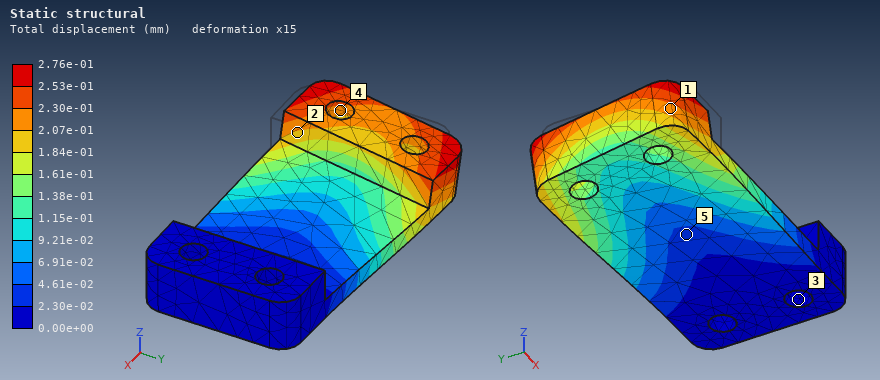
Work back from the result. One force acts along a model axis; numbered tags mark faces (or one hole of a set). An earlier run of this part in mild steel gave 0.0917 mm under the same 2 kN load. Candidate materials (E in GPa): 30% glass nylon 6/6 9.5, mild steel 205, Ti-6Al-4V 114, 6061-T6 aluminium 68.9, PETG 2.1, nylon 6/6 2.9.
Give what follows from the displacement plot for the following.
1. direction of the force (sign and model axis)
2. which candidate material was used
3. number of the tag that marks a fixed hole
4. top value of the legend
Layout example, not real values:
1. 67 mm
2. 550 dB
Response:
1. +Y
2. 6061-T6 aluminium
3. 3
4. 2.76e-01 mm
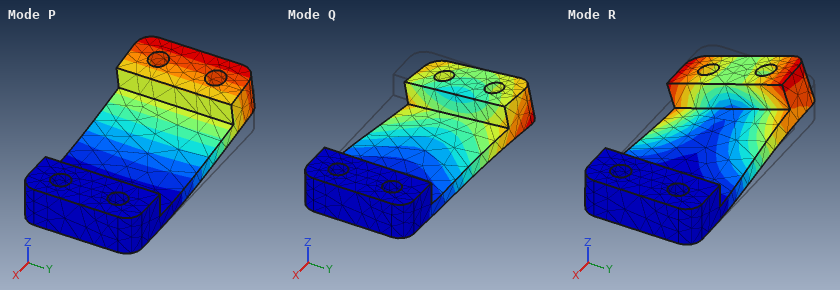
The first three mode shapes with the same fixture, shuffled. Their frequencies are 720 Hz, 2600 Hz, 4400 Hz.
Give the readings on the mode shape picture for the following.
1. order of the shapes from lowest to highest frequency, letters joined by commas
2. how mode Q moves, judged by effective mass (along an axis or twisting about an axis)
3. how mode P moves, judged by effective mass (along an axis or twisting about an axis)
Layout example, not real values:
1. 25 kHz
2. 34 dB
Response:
1. P, R, Q
2. along Y
3. along Z
